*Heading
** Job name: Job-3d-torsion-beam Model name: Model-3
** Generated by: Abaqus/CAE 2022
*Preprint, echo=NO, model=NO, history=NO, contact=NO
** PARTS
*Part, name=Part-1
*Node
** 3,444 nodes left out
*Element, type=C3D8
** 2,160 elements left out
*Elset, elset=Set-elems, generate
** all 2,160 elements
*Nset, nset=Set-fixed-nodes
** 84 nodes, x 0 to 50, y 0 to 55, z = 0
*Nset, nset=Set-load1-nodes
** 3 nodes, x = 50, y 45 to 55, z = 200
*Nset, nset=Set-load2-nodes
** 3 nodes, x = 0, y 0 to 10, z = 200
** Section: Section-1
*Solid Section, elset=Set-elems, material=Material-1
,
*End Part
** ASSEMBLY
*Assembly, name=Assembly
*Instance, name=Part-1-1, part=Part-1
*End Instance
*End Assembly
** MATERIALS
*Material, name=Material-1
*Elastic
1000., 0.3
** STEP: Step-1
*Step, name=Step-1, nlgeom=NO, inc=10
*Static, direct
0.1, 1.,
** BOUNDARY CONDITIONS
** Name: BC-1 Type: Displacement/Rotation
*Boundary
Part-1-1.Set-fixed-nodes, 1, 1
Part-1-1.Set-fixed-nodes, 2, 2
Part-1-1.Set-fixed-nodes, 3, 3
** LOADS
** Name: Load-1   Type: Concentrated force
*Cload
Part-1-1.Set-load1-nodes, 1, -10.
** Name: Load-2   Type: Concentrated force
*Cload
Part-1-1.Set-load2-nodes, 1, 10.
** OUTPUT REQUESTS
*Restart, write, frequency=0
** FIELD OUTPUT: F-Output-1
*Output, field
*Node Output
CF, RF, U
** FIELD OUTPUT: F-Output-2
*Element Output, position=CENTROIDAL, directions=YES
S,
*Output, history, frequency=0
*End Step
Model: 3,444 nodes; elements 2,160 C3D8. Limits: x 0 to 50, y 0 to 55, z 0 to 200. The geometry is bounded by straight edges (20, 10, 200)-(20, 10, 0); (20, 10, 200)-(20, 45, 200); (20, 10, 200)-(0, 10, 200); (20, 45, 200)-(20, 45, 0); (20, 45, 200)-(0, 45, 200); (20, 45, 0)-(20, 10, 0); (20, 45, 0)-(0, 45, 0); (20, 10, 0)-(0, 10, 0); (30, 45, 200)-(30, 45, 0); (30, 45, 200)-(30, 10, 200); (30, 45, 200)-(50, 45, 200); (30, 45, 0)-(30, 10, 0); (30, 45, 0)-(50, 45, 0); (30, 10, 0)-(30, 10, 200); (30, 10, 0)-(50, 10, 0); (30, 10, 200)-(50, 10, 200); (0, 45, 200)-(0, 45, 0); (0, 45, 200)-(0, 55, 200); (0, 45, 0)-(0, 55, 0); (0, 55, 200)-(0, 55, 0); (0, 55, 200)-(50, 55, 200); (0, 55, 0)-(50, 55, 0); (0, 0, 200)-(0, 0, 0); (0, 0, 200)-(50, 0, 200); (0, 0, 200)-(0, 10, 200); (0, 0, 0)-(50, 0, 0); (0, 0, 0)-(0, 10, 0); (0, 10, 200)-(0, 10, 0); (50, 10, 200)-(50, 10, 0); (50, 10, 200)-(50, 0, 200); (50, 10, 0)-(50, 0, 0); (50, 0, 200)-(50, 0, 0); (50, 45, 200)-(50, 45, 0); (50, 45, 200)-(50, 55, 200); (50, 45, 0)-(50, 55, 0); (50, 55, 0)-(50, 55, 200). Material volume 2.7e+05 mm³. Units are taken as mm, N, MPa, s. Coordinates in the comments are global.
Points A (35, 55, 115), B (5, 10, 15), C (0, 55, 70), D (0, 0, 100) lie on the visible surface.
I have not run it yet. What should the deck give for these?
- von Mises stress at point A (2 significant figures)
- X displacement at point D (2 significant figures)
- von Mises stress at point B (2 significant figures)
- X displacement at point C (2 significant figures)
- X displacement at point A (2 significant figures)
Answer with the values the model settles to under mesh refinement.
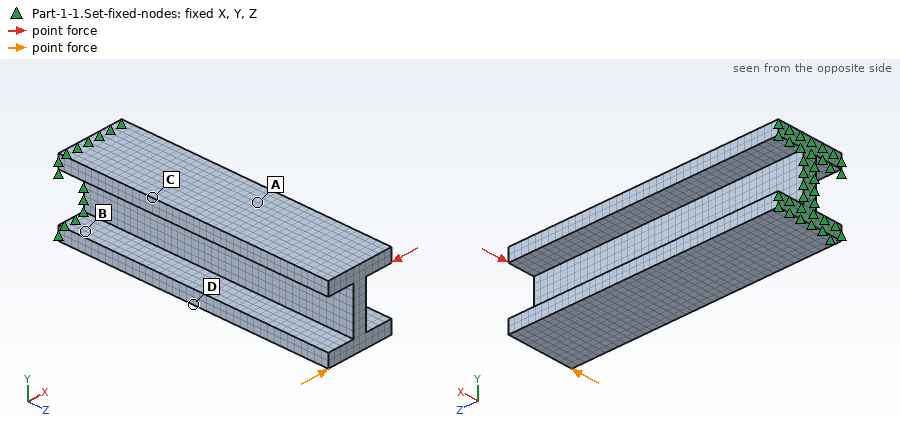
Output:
0.44 MPa
0.10 mm
0.45 MPa
-0.060 mm
-0.13 mm
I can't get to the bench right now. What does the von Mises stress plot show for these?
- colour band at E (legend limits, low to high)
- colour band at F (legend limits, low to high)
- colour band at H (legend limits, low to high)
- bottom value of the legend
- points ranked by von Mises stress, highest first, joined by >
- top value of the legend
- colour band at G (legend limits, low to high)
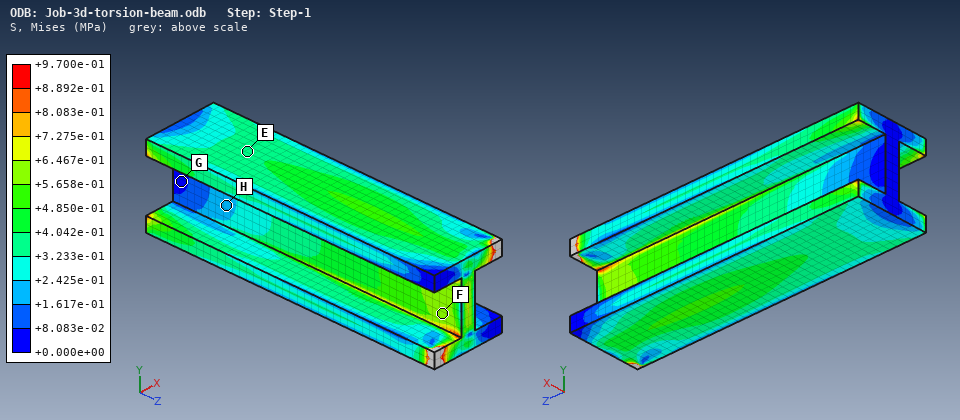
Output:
+3.233e-01 to +4.042e-01 MPa
+5.658e-01 to +6.467e-01 MPa
+1.617e-01 to +2.425e-01 MPa
+0.000e+00 MPa
F > E > H > G
+9.700e-01 MPa
+0.000e+00 to +8.083e-02 MPa
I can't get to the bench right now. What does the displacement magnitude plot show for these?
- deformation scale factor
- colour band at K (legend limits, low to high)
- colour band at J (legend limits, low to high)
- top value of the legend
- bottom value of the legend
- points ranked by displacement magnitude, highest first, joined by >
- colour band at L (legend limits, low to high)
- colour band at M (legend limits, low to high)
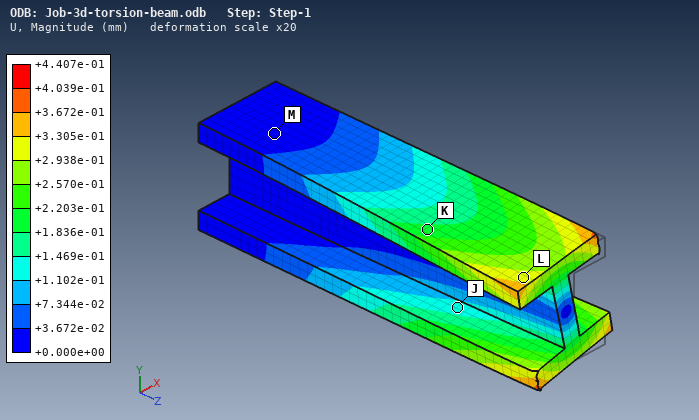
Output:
20
+1.836e-01 to +2.203e-01 mm
+1.102e-01 to +1.469e-01 mm
+4.407e-01 mm
+0.000e+00 mm
L > K > J > M
+2.938e-01 to +3.305e-01 mm
+0.000e+00 to +3.672e-02 mm
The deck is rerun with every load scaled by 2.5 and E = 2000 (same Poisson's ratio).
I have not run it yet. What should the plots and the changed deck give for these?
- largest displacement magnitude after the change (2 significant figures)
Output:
0.55 mm
